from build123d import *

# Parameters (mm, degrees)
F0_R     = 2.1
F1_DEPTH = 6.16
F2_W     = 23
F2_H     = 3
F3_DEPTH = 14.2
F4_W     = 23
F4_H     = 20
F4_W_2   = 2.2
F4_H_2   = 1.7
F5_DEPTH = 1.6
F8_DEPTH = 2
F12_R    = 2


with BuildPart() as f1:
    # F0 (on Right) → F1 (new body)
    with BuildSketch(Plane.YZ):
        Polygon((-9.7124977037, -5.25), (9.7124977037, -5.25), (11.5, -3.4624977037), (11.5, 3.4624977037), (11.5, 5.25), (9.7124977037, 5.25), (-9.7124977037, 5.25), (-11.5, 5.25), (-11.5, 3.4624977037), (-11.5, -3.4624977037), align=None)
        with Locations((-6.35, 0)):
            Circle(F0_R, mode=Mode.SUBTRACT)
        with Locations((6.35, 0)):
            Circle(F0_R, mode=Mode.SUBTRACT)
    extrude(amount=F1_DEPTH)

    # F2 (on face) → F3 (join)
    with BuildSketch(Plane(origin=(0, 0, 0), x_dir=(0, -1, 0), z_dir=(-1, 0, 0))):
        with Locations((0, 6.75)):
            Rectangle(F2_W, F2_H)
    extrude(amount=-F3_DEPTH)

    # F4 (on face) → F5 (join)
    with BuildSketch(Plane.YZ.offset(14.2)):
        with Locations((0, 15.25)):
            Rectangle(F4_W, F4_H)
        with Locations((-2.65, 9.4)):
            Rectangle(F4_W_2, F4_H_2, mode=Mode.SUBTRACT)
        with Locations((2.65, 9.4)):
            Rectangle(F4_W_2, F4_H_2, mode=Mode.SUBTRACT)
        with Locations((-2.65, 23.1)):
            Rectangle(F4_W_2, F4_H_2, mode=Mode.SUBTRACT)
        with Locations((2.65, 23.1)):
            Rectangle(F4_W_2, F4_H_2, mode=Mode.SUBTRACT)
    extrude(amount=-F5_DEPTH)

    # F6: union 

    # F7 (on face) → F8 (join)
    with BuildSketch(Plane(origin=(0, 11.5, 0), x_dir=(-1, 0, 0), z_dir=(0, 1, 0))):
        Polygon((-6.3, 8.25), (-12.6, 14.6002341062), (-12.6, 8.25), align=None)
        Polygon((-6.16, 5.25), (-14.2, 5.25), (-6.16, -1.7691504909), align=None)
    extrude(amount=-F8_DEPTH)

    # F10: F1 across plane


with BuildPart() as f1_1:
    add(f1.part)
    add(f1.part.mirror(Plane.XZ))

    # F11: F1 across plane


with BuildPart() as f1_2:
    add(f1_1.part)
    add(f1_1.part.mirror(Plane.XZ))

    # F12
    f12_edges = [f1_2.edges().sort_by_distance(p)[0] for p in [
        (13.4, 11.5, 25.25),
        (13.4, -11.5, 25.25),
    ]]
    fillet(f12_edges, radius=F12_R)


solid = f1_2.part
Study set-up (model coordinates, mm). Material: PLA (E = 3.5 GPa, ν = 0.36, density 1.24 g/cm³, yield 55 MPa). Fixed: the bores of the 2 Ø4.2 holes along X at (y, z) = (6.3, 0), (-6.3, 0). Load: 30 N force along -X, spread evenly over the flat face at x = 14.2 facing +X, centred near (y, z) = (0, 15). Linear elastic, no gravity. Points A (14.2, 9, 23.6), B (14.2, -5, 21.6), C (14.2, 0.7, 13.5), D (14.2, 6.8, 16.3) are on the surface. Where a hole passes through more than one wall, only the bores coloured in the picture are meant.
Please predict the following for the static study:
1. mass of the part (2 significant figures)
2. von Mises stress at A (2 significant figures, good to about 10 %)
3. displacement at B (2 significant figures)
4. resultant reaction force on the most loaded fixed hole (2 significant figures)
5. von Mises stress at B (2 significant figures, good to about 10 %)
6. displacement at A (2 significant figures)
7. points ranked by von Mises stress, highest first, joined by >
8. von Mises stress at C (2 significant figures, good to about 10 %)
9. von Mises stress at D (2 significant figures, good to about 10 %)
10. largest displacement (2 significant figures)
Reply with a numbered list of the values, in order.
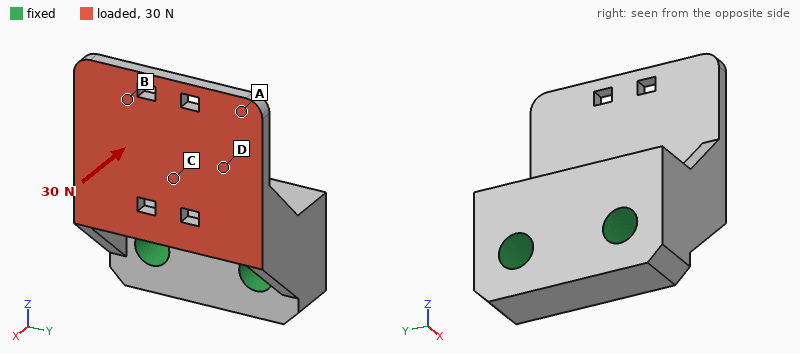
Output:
1. 3.8 g
2. 1.2 MPa
3. 0.30 mm
4. 16 N
5. 3.3 MPa
6. 0.33 mm
7. D > C > B > A
8. 4.7 MPa
9. 6.7 MPa
10. 0.43 mm
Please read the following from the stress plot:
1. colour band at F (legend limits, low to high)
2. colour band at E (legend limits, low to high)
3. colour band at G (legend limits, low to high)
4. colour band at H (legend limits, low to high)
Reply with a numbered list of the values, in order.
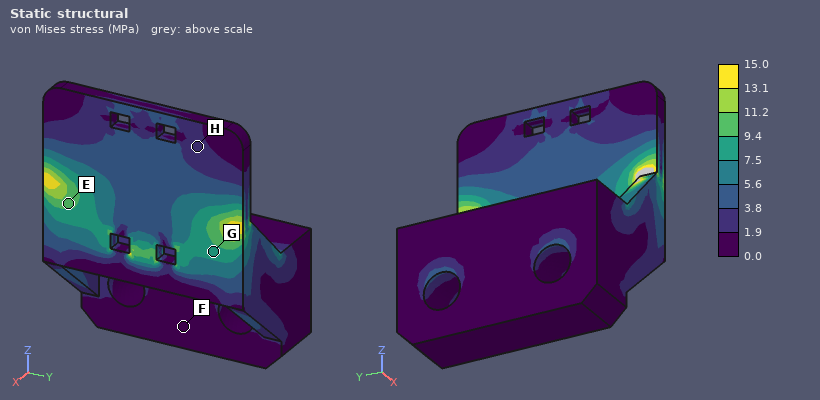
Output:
1. 0.0 to 1.9 MPa
2. 9.4 to 11.2 MPa
3. 7.5 to 9.4 MPa
4. 1.9 to 3.8 MPa
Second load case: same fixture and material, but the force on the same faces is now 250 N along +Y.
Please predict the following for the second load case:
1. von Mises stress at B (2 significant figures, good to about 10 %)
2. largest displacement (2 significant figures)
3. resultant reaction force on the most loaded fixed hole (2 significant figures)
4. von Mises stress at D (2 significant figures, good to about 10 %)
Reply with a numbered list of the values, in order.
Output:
1. 5.4 MPa
2. 0.24 mm
3. 290 N
4. 6.5 MPa
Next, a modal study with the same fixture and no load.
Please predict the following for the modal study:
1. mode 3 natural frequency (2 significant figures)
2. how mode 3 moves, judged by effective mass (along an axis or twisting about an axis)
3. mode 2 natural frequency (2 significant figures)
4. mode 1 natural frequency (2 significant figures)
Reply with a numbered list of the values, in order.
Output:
1. 5700 Hz
2. along Z
3. 3500 Hz
4. 1800 Hz
